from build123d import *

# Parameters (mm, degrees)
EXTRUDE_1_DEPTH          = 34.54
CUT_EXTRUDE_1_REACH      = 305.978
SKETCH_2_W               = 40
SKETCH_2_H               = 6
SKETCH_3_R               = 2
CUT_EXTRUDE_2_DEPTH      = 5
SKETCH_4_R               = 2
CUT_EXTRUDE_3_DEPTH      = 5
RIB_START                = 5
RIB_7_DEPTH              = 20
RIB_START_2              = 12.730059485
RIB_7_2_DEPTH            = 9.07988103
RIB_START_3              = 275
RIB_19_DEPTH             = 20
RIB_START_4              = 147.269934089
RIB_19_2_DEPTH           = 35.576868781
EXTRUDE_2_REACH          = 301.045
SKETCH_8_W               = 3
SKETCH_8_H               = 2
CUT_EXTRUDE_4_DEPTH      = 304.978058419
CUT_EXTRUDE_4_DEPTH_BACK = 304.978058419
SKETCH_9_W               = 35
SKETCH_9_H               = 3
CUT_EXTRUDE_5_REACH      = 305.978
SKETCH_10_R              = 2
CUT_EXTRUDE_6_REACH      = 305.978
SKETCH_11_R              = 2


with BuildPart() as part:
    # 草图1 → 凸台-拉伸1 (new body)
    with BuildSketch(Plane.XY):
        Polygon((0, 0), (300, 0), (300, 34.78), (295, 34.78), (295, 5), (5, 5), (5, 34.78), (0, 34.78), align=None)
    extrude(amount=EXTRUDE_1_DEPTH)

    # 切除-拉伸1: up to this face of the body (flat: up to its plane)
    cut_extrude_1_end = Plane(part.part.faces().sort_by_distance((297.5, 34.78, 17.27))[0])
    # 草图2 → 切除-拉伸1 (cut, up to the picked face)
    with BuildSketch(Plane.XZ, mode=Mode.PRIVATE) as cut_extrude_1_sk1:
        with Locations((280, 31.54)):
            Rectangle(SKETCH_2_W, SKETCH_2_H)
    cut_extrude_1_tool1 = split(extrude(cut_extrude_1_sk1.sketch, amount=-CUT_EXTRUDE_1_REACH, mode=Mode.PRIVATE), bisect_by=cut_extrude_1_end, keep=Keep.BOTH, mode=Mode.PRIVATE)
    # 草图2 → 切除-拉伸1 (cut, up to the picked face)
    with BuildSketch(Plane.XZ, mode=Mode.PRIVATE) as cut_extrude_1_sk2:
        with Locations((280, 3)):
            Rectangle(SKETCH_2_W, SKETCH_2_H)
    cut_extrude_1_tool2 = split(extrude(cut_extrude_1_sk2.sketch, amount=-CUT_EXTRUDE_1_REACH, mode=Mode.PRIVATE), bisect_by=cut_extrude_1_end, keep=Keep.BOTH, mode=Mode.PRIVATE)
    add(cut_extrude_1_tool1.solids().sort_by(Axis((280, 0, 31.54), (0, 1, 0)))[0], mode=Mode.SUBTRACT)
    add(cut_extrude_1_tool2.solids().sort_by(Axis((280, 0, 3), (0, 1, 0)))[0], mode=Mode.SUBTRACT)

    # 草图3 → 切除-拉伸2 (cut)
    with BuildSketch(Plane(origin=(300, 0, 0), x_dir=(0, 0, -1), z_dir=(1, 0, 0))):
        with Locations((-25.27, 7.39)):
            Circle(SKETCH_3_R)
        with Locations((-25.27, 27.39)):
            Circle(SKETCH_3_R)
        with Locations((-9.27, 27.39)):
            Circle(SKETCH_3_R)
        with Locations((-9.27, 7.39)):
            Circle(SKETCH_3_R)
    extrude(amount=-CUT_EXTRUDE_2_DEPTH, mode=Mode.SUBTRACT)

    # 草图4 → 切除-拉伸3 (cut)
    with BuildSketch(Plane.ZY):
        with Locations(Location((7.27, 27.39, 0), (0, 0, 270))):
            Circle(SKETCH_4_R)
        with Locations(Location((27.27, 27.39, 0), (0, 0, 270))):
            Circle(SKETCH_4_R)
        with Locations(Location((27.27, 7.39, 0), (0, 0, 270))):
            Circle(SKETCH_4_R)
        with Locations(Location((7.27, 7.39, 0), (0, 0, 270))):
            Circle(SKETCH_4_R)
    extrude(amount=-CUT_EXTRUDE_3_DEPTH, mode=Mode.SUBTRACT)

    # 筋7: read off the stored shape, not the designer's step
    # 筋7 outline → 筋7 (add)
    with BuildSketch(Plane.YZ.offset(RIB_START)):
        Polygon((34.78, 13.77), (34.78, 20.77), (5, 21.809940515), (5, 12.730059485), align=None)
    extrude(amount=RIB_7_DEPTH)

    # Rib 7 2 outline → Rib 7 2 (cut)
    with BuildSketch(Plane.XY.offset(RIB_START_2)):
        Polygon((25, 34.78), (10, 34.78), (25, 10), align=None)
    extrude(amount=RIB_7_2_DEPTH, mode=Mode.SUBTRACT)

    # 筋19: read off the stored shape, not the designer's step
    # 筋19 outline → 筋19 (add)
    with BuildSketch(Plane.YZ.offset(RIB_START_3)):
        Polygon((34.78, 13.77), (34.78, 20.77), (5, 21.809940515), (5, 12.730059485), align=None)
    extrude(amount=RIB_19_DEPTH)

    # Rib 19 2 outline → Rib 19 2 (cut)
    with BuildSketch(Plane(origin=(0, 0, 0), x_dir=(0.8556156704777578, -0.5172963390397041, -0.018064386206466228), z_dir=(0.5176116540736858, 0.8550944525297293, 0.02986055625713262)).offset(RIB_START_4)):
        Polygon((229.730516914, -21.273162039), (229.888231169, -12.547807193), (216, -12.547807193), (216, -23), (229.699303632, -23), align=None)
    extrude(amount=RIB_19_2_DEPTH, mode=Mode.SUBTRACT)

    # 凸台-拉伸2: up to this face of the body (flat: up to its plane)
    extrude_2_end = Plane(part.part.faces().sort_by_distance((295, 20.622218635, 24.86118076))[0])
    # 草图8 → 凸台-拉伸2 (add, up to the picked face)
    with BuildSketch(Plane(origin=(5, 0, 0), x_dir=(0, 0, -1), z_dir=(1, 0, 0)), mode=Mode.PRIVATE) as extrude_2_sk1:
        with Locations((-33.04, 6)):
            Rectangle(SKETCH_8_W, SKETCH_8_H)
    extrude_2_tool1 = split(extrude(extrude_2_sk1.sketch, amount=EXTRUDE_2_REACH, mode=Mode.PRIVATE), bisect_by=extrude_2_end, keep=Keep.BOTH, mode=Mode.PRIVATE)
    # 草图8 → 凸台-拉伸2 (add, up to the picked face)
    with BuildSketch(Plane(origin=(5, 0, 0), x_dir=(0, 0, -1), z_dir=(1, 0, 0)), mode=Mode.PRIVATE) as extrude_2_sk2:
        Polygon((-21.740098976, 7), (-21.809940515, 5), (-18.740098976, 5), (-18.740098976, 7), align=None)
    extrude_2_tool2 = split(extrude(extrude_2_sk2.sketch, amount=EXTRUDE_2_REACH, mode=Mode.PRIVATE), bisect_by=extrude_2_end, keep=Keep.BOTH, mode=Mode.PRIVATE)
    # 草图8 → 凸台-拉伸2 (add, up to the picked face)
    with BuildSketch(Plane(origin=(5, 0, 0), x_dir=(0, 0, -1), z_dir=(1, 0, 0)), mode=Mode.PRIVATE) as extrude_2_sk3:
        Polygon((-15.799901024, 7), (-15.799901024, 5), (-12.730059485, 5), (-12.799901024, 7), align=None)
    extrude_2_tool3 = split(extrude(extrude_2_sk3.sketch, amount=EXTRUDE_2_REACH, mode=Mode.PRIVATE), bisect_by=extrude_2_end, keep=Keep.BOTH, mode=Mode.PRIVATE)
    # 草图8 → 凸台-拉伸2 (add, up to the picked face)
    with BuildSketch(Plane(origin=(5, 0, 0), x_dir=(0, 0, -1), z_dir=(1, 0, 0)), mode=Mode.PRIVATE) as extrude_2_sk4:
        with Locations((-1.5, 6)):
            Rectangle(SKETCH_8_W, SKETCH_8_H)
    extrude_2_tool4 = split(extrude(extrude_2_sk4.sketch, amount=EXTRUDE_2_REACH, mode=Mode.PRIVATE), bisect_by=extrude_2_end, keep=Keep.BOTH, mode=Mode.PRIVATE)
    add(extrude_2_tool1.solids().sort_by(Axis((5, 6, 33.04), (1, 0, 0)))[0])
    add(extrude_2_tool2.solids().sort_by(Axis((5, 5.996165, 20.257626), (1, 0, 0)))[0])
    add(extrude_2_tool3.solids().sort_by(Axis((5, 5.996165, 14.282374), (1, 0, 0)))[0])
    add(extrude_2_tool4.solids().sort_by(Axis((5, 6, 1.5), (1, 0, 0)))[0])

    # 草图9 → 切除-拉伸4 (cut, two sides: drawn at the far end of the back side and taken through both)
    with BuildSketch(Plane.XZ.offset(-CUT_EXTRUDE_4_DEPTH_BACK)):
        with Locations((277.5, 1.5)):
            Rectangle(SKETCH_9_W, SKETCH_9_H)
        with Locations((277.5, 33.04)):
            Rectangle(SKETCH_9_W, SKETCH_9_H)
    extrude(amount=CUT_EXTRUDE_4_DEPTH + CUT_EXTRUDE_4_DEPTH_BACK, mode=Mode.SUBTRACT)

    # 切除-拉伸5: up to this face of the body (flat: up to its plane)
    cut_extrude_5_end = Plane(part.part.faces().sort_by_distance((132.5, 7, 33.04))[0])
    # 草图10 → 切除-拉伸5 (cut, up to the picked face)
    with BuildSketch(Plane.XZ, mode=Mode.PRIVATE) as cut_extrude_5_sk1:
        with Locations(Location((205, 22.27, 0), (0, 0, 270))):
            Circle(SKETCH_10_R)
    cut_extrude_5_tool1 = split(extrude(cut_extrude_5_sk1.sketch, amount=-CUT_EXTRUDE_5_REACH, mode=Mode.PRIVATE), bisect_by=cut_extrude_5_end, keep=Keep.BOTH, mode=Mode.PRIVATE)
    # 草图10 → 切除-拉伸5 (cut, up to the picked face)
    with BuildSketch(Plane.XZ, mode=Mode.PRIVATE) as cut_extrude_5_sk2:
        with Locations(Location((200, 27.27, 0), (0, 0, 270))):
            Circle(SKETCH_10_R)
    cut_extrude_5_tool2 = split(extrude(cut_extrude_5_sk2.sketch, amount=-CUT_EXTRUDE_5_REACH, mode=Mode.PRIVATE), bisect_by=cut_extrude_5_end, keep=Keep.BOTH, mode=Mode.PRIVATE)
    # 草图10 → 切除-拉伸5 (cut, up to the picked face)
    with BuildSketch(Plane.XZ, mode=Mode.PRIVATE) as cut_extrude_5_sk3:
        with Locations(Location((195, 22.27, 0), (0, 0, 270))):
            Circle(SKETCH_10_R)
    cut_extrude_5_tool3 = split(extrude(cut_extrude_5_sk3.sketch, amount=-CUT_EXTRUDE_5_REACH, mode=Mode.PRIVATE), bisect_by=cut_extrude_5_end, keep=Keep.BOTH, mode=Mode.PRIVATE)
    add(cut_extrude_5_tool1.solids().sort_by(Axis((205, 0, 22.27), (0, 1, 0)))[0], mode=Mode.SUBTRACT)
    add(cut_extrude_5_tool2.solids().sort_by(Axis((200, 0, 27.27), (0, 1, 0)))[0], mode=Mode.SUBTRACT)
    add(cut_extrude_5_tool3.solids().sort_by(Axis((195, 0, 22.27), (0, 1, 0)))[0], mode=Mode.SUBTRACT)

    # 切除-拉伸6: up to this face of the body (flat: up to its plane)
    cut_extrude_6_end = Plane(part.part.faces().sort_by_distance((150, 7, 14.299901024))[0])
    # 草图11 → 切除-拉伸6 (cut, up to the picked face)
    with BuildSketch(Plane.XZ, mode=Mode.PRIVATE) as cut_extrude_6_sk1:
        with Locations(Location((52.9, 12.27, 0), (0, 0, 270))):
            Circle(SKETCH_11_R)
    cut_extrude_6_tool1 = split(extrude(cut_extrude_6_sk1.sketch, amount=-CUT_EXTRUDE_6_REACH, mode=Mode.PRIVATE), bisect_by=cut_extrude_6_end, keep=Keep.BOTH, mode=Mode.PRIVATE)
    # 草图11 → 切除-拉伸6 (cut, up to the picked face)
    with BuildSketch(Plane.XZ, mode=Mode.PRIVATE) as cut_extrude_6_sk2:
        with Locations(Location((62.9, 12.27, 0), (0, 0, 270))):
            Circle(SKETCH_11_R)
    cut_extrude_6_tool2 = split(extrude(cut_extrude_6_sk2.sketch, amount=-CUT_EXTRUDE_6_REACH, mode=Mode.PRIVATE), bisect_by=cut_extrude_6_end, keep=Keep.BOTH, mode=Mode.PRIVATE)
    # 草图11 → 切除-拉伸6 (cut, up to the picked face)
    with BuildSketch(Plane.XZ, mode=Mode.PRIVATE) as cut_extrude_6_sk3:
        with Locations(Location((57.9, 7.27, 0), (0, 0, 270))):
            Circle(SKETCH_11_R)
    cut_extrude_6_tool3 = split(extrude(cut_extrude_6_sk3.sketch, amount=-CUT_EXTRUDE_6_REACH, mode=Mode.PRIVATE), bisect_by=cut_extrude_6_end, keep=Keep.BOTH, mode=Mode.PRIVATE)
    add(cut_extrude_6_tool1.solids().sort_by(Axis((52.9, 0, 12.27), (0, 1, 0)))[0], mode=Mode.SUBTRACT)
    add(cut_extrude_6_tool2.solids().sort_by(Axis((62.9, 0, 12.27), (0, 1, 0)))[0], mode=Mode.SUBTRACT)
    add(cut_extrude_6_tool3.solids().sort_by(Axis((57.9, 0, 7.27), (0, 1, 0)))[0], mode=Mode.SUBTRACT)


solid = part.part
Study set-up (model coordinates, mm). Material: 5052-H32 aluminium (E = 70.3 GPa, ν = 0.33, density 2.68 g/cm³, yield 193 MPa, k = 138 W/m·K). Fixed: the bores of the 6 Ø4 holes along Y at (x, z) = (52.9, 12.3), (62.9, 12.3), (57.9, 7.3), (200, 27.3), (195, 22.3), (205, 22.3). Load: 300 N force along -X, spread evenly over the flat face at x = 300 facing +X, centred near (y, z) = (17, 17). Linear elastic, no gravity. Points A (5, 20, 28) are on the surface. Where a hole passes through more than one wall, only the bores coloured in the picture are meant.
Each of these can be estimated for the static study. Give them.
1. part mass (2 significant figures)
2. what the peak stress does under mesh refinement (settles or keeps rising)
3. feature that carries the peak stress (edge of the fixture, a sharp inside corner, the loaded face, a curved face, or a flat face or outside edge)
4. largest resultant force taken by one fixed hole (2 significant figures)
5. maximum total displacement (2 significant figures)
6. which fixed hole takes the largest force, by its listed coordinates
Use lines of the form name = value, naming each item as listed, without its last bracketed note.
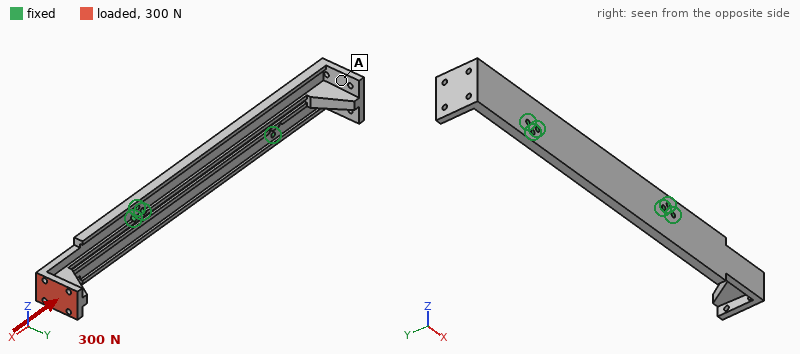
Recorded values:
part mass = 190 g
what the peak stress does under mesh refinement = keeps rising
feature that carries the peak stress = edge of the fixture
largest resultant force taken by one fixed hole = 270 N
maximum total displacement = 0.58 mm
which fixed hole takes the largest force, by its listed coordinates = (205, 22.3)
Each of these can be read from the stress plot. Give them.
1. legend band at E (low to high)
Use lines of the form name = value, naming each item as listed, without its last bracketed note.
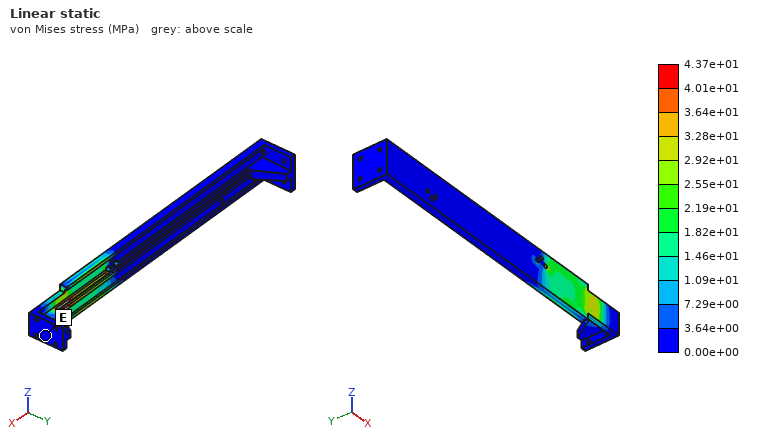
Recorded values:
legend band at E = 0.00e+00 to 3.64e+00 MPa
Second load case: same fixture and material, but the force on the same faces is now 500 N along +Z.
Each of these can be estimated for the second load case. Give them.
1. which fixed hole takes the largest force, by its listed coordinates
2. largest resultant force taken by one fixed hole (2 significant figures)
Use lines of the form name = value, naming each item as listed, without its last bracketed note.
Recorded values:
which fixed hole takes the largest force, by its listed coordinates = (205, 22.3)
largest resultant force taken by one fixed hole = 1.9 kN
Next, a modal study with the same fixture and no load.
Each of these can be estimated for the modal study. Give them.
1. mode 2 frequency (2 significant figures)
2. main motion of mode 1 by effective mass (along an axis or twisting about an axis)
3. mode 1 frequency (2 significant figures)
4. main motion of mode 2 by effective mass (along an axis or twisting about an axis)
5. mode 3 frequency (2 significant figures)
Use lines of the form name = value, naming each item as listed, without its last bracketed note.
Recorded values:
mode 2 frequency = 890 Hz
main motion of mode 1 by effective mass = along Y
mode 1 frequency = 400 Hz
main motion of mode 2 by effective mass = along Y
mode 3 frequency = 1100 Hz
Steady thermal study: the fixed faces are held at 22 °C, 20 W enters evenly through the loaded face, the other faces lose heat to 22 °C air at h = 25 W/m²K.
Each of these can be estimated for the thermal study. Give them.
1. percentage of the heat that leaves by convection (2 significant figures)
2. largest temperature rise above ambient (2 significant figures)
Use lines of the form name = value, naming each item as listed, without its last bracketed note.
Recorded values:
percentage of the heat that leaves by convection = 38 %
largest temperature rise above ambient = 62 K
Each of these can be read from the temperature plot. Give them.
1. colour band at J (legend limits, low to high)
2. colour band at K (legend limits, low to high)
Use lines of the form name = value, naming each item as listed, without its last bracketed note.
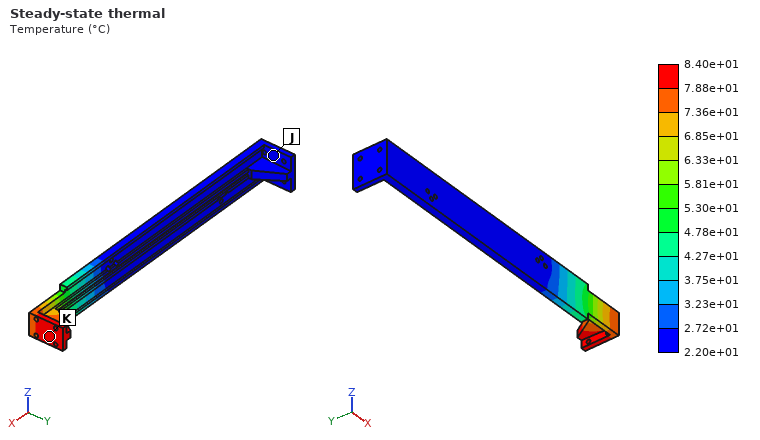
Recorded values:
colour band at J = 2.20e+01 to 2.72e+01 °C
colour band at K = 7.88e+01 to 8.40e+01 °C
